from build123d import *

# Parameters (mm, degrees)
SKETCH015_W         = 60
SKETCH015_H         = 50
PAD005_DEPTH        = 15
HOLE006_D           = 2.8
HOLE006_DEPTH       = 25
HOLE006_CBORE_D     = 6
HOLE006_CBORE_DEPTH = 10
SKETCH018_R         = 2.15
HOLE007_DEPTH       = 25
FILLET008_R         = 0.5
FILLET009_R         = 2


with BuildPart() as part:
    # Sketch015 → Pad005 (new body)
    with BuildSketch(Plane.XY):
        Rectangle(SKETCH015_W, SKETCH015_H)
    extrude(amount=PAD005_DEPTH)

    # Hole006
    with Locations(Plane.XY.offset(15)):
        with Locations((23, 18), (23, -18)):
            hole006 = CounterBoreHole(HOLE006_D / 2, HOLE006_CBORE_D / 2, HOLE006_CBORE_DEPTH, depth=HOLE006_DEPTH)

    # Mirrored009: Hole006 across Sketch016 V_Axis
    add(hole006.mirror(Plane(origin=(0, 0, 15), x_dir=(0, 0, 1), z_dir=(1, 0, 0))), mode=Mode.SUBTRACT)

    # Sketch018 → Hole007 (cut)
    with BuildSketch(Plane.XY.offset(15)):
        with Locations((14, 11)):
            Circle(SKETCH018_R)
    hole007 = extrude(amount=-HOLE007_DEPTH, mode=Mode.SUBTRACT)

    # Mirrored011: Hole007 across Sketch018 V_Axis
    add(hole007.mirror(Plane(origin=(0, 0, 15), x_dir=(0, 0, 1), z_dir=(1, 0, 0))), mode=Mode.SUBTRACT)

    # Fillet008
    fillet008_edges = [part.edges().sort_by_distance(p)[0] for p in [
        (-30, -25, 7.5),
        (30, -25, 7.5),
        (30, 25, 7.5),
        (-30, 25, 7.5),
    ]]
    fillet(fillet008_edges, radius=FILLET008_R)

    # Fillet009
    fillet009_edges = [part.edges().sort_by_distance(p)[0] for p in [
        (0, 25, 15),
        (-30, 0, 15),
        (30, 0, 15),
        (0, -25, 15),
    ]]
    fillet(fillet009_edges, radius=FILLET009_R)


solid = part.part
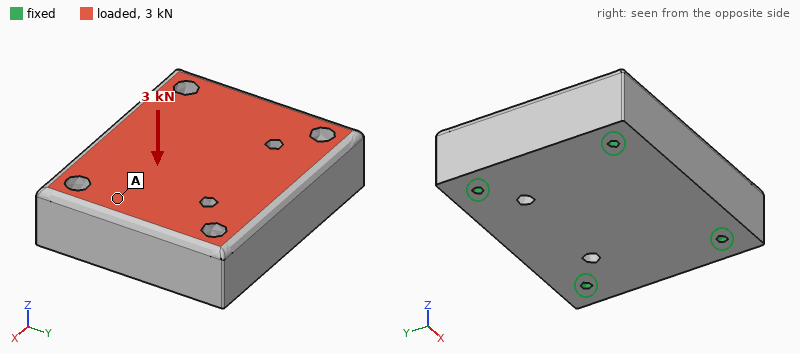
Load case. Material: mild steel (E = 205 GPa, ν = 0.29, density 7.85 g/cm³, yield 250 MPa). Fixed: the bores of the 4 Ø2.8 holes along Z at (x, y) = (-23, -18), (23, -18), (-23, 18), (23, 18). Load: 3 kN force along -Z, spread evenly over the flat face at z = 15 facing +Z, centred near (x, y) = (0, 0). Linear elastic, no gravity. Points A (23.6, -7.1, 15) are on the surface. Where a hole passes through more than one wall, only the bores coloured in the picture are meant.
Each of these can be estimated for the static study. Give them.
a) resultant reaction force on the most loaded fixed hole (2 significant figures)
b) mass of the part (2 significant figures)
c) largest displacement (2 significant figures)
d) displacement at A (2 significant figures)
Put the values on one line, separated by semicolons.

840 N; 340 g; 1.6 µm; 0.91 µm
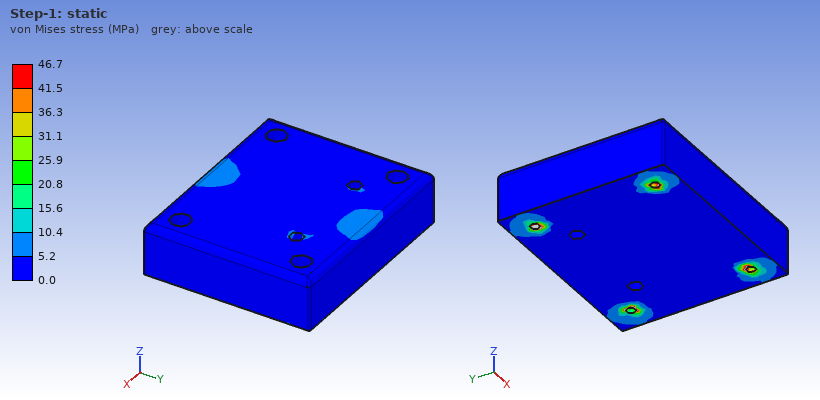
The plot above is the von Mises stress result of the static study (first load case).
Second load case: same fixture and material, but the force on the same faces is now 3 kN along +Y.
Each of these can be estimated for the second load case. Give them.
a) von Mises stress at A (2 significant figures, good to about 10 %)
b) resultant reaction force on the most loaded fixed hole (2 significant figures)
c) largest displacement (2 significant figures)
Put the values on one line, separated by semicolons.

4.0 MPa; 940 N; 1.6 µm
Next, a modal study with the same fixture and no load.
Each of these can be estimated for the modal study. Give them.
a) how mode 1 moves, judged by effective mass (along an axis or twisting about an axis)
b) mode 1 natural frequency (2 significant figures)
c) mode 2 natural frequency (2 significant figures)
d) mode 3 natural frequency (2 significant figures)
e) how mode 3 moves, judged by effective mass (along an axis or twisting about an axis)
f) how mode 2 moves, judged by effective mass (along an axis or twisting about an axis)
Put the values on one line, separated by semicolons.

along Z; 14 kHz; 17 kHz; 19 kHz; along X; along Y
